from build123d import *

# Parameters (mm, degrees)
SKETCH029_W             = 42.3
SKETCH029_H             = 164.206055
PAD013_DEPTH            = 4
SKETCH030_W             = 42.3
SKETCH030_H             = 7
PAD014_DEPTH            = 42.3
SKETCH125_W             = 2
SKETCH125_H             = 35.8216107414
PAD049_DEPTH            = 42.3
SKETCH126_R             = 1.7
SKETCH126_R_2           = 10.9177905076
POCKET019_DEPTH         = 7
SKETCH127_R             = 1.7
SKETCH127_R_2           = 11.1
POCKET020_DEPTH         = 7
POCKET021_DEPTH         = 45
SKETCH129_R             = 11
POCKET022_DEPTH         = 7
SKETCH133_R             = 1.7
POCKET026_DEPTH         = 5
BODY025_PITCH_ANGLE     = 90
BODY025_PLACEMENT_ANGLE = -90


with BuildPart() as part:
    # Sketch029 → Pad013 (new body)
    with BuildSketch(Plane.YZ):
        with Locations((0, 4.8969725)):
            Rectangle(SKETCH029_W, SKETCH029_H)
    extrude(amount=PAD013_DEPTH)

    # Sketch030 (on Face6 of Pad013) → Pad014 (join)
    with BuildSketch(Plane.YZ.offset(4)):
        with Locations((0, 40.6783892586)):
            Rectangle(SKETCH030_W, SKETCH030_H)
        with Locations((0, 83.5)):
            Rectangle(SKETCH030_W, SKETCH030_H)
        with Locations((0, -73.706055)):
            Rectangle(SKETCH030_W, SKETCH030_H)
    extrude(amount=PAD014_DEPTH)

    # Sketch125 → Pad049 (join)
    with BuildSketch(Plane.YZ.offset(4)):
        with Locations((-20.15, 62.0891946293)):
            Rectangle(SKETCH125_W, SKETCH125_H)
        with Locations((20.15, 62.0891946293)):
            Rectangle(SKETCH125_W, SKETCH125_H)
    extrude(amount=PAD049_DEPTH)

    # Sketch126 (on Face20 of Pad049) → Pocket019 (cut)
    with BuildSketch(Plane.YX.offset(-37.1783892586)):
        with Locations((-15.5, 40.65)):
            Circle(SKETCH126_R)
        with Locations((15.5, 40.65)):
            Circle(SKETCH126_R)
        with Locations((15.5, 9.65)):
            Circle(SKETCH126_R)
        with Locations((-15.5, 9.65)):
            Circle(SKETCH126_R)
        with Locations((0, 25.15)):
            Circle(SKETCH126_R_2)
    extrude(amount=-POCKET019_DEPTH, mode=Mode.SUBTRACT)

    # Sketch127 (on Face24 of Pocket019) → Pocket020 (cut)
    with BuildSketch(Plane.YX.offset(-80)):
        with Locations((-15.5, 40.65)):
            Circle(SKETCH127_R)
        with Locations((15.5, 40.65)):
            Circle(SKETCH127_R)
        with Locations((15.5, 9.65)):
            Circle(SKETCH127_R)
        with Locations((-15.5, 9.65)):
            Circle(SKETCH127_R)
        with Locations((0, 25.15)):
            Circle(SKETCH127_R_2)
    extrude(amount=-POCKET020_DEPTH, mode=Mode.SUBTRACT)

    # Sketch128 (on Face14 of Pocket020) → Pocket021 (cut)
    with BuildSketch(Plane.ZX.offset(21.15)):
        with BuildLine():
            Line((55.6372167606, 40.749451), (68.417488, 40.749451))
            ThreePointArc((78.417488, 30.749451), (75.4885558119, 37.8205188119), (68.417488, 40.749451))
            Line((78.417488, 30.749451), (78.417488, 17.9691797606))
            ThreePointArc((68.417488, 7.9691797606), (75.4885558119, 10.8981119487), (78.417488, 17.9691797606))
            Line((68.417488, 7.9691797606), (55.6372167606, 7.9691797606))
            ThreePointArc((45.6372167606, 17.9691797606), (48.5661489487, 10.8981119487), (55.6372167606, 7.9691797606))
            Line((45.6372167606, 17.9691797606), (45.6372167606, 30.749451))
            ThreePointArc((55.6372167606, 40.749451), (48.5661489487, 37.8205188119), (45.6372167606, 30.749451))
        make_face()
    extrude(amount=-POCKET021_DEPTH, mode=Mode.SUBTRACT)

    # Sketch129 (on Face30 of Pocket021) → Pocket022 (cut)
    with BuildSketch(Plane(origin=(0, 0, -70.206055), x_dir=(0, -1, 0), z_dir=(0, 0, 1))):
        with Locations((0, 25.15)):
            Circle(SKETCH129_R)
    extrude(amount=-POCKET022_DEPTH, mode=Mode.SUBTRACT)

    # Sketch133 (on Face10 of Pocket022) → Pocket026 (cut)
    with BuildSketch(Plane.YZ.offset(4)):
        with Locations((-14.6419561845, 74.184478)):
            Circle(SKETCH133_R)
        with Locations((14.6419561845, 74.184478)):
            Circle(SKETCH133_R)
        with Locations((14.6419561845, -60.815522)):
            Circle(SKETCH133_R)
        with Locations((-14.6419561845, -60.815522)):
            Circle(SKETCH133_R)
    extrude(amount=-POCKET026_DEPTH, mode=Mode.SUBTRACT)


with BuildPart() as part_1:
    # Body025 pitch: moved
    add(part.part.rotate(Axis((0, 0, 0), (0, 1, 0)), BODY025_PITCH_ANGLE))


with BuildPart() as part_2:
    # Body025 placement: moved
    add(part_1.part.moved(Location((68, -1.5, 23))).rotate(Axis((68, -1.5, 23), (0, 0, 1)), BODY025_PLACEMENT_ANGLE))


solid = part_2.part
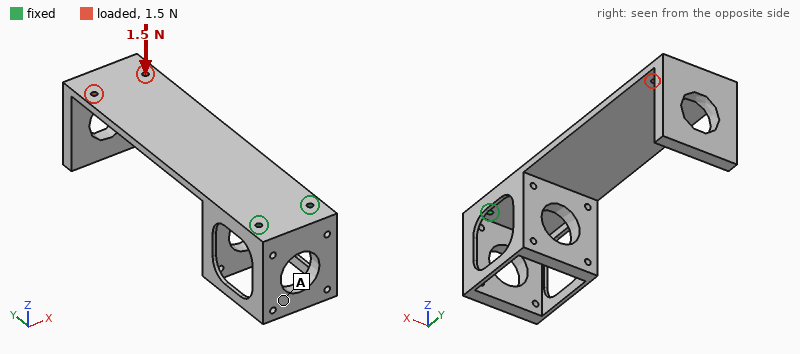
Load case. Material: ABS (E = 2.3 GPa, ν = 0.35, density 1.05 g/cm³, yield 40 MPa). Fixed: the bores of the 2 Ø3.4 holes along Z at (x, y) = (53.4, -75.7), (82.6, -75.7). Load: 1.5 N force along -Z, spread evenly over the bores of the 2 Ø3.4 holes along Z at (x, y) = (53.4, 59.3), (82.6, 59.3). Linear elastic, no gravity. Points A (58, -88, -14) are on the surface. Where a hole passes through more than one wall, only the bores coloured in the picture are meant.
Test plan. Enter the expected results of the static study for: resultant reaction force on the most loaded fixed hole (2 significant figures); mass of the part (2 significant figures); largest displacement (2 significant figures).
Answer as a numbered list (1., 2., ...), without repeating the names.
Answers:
1. 1.2 N
2. 62 g
3. 1.7 mm
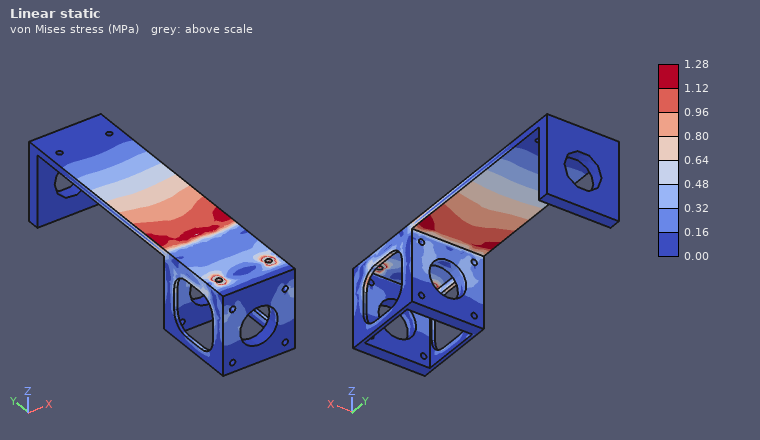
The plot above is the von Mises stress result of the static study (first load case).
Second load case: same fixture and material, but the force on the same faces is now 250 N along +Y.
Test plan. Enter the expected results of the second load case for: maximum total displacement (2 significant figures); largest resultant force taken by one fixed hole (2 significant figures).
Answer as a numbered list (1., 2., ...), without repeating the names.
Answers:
1. 0.19 mm
2. 130 N
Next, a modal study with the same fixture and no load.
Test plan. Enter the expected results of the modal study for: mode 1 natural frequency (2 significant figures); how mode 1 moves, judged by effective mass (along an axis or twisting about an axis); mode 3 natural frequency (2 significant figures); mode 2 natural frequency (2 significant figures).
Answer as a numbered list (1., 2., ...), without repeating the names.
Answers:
1. 36 Hz
2. along Z
3. 170 Hz
4. 130 Hz
